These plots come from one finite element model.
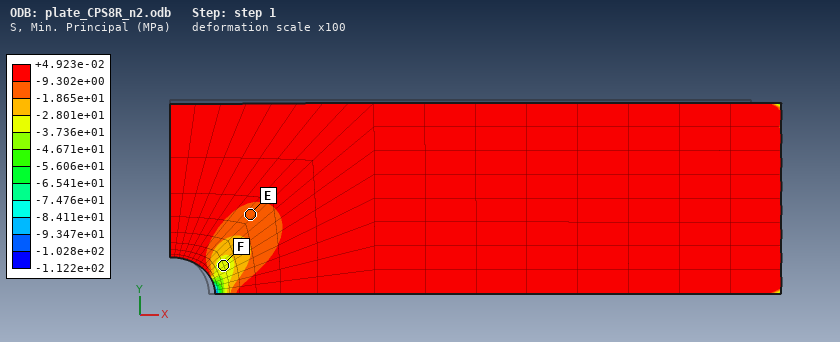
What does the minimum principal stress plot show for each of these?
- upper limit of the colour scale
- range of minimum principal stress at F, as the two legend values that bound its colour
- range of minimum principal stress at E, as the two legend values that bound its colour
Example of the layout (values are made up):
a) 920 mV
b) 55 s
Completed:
a) +4.923e-02 MPa
b) -3.736e+01 to -2.801e+01 MPa
c) -1.865e+01 to -9.302e+00 MPa
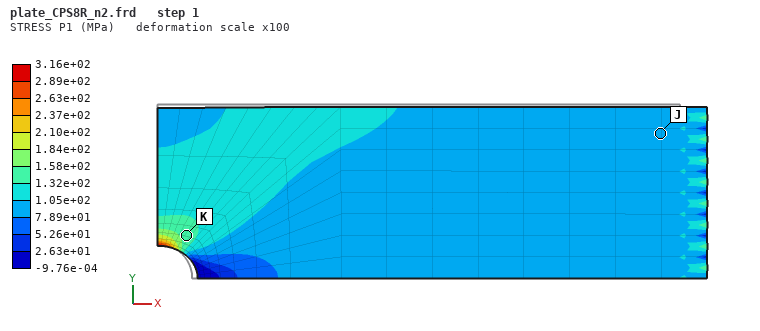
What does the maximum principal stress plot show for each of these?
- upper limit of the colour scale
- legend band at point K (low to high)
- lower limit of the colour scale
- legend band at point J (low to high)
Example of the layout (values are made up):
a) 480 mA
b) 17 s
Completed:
a) 3.16e+02 MPa
b) 1.32e+02 to 1.58e+02 MPa
c) -9.76e-04 MPa
d) 7.89e+01 to 1.05e+02 MPa
